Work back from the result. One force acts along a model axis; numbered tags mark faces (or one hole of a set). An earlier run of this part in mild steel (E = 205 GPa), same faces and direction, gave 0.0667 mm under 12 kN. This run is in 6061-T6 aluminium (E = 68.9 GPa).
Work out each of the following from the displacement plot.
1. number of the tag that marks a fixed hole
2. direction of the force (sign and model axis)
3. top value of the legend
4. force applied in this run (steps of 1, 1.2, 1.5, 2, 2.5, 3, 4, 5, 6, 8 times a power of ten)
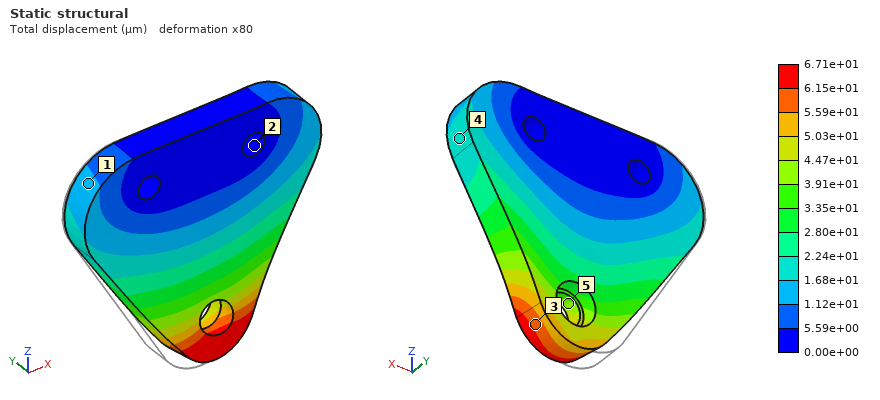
2
+X
6.71e+01 µm
4 kN
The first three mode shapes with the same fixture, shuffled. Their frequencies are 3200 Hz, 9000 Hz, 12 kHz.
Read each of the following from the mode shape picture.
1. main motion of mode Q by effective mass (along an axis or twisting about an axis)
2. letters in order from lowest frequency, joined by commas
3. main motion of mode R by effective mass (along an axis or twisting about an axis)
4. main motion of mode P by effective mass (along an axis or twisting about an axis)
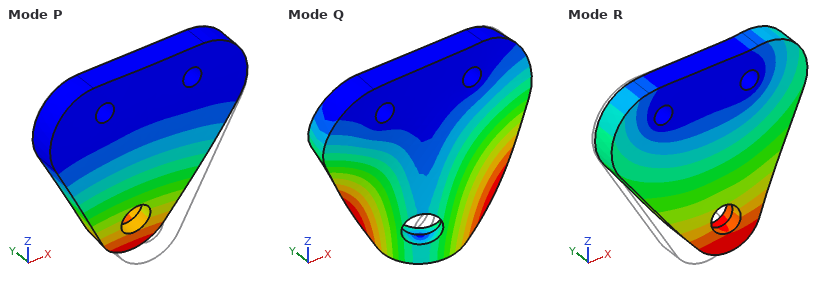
twisting about Z
P, Q, R
along X
along Y
